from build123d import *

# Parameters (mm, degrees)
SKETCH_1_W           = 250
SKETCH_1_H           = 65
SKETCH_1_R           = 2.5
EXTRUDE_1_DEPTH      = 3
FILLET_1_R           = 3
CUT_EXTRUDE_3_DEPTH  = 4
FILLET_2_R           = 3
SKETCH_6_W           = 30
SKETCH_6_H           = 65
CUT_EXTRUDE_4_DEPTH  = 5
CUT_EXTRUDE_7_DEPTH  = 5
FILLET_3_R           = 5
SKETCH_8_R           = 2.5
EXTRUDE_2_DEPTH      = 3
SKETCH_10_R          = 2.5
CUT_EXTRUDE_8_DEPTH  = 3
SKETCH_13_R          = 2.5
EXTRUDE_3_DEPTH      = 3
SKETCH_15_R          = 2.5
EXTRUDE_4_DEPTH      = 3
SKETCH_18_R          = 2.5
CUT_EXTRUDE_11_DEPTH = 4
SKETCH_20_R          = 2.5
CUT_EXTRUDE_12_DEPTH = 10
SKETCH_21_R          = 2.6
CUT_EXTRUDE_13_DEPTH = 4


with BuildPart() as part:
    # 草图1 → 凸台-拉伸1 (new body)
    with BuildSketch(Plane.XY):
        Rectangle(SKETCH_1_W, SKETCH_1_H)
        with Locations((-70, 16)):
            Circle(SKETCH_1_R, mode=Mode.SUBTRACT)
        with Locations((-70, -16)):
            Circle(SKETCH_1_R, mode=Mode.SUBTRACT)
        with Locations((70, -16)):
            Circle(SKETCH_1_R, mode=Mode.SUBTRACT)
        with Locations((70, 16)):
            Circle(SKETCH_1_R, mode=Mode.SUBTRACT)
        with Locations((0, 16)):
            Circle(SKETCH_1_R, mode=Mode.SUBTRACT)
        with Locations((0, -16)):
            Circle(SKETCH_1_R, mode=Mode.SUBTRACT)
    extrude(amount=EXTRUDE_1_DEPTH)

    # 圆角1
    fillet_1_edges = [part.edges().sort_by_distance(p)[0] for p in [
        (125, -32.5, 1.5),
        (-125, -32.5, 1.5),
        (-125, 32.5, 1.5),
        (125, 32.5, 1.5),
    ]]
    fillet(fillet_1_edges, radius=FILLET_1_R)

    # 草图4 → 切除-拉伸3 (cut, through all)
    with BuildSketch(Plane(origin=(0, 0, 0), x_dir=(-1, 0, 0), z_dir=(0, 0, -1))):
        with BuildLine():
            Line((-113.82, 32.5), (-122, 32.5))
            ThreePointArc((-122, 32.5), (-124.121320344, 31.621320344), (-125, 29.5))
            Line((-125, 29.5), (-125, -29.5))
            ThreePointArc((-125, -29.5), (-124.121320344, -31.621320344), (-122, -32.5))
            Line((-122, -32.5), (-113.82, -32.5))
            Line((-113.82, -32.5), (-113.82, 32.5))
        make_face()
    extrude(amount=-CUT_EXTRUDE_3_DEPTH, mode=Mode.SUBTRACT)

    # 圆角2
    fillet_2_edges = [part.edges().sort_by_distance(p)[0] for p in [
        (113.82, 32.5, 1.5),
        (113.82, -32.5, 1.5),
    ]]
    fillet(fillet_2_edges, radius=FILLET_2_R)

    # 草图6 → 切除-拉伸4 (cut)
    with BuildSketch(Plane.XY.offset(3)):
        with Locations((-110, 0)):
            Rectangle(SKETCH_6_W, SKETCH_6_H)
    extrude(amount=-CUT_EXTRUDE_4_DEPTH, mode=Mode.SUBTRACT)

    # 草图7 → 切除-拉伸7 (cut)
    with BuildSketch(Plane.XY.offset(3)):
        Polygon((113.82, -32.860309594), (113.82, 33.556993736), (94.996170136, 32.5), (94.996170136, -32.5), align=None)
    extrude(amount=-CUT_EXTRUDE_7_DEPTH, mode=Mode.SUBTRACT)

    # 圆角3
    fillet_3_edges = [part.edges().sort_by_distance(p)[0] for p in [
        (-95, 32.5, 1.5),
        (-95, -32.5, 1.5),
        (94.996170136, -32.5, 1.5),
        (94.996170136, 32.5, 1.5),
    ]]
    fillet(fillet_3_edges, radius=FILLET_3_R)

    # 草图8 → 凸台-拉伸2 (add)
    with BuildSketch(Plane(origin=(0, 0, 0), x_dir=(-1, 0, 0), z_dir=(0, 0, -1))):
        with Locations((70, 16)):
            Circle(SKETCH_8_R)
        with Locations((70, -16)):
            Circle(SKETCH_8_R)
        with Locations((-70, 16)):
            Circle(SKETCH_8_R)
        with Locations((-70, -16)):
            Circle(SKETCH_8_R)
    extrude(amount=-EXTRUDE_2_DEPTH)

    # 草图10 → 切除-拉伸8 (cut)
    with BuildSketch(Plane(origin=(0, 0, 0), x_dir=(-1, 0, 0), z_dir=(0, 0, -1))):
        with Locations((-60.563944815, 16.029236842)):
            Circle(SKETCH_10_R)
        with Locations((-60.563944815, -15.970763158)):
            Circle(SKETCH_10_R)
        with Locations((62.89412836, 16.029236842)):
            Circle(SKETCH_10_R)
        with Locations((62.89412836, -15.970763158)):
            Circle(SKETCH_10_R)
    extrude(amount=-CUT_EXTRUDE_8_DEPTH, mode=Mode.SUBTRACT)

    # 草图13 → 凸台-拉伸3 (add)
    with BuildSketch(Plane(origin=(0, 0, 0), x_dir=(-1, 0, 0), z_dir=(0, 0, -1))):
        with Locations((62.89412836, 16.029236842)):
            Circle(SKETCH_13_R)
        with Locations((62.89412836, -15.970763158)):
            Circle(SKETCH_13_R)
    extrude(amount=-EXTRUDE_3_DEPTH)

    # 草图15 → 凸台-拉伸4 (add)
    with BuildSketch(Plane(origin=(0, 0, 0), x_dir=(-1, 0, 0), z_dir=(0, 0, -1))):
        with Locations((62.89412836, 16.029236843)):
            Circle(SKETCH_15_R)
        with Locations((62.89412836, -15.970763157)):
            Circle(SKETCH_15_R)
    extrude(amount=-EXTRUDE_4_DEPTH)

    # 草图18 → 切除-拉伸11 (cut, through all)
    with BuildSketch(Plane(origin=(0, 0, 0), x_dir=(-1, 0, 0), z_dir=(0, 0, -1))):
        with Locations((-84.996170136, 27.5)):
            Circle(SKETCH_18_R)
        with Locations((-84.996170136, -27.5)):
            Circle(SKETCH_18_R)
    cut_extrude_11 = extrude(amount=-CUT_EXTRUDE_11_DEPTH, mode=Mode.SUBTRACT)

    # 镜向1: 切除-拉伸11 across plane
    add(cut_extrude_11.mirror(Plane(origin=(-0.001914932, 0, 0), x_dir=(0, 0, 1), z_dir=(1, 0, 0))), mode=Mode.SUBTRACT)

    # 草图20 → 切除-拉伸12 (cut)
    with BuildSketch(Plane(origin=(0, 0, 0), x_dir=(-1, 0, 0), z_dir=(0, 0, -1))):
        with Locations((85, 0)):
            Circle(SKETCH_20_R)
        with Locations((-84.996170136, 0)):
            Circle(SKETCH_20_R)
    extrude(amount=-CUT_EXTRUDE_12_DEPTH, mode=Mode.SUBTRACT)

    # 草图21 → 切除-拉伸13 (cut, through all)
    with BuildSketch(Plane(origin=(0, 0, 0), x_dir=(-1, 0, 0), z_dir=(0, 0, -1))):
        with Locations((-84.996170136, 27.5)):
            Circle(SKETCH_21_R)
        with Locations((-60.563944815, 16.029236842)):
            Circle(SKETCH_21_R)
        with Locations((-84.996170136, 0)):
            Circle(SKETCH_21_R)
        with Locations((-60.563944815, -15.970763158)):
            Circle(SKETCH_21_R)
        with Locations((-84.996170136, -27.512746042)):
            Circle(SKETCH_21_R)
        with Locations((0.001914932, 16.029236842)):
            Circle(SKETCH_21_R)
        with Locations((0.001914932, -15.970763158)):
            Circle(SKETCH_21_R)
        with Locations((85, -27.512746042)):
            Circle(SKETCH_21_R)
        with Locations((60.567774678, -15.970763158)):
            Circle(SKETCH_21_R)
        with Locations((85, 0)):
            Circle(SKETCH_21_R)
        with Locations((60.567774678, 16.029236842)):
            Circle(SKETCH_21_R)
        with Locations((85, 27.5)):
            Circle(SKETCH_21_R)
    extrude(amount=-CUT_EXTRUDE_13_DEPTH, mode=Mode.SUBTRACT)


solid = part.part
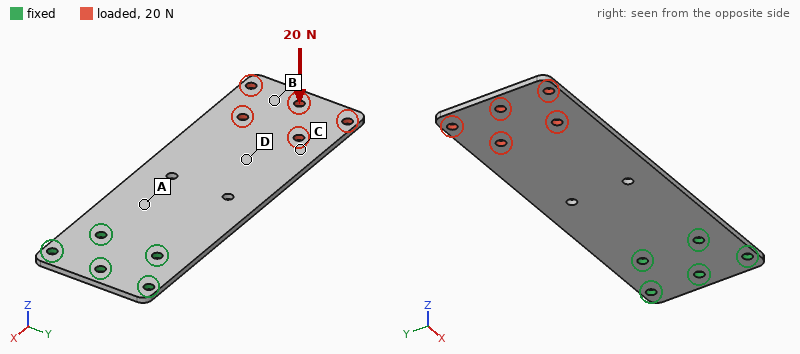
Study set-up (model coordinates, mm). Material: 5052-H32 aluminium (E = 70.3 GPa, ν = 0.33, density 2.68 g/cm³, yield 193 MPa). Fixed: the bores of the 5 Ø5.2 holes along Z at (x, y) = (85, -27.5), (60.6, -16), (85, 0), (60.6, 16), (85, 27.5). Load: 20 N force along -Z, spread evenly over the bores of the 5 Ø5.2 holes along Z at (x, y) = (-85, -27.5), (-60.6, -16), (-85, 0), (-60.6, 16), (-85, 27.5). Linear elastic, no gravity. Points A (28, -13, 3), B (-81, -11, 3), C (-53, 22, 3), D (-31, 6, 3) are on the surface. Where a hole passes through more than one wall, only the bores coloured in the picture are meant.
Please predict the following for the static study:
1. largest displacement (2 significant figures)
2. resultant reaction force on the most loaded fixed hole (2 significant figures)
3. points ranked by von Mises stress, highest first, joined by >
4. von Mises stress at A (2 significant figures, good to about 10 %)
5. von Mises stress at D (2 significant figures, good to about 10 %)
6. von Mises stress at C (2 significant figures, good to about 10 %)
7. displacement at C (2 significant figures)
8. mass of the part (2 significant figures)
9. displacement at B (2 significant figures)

1.9 mm
28 N
A > D > C > B
20 MPa
9.0 MPa
5.0 MPa
1.2 mm
97 g
1.7 mm
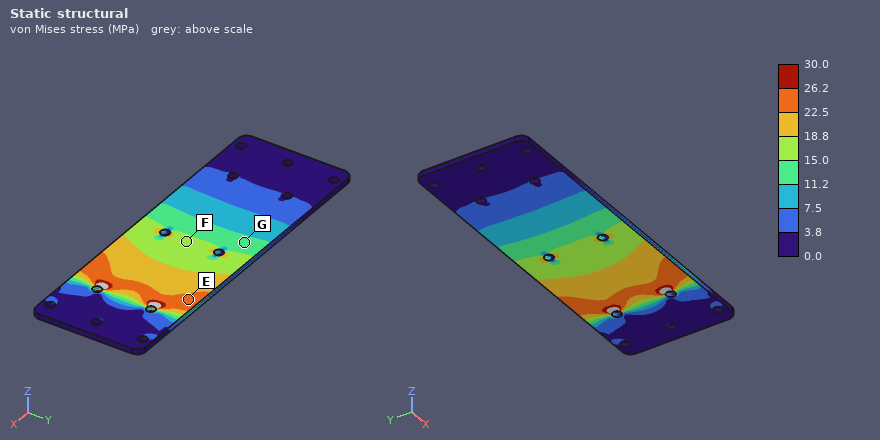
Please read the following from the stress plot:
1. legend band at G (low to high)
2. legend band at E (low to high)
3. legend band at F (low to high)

11.2 to 15.0 MPa
22.5 to 26.2 MPa
15.0 to 18.8 MPa
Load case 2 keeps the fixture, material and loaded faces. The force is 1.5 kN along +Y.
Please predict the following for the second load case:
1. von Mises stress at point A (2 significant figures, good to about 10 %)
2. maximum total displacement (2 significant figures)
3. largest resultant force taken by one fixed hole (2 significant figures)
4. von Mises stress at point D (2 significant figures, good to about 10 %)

36 MPa
0.44 mm
3.7 kN
20 MPa
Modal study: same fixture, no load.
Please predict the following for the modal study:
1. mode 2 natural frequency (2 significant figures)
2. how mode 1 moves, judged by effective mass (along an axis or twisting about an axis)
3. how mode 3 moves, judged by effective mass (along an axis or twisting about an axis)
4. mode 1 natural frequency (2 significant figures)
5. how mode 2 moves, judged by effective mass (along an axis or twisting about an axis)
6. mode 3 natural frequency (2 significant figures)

510 Hz
along Z
along Z
110 Hz
twisting about X
650 Hz
